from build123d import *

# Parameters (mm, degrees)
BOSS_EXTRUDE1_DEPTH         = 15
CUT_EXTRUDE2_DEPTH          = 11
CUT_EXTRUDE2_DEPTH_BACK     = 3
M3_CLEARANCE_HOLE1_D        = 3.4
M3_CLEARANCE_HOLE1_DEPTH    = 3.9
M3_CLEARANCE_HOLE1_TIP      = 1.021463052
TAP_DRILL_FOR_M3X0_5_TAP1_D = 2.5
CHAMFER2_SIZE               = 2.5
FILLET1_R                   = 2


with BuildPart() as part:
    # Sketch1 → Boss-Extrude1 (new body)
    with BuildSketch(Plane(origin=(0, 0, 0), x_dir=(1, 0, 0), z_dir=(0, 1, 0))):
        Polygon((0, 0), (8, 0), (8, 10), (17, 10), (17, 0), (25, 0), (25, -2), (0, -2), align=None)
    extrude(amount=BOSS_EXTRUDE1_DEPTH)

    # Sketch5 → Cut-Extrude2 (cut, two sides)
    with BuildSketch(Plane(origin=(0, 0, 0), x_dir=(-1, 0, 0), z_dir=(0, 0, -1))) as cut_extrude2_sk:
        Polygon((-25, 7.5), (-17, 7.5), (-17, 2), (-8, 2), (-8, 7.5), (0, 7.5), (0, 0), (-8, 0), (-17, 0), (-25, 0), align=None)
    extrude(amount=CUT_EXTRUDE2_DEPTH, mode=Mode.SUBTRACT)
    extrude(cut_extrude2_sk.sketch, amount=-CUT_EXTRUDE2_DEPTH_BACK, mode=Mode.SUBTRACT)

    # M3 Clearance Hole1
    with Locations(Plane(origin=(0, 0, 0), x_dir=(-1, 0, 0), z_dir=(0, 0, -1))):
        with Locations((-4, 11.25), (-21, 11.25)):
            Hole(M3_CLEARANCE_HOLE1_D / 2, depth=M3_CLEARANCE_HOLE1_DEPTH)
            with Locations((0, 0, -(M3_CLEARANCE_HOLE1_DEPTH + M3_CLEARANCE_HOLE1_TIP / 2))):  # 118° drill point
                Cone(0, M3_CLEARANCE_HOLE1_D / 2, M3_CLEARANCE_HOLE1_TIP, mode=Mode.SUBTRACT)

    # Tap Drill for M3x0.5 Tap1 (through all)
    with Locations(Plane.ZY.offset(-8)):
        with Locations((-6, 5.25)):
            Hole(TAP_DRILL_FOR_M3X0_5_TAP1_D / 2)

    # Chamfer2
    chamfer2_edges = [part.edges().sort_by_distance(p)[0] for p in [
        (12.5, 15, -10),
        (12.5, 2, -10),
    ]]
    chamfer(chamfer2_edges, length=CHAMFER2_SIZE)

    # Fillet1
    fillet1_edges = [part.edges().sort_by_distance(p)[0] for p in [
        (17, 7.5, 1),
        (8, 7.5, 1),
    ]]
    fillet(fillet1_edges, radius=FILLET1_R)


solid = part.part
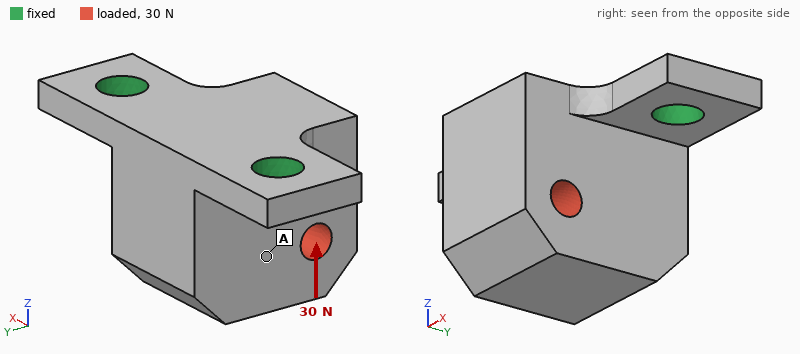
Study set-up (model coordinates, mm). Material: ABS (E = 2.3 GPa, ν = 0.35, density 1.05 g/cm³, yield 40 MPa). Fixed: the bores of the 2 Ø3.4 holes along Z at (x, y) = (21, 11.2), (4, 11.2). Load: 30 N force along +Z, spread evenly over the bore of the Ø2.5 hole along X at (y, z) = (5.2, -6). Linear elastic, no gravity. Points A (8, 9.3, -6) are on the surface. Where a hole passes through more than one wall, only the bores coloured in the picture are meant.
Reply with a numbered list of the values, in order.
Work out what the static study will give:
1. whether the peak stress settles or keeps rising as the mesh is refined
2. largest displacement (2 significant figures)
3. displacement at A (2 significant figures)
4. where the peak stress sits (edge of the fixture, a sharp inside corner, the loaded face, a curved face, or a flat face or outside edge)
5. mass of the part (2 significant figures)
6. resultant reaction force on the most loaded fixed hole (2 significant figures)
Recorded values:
1. keeps rising
2. 0.17 mm
3. 0.098 mm
4. edge of the fixture
5. 1.6 g
6. 16 N
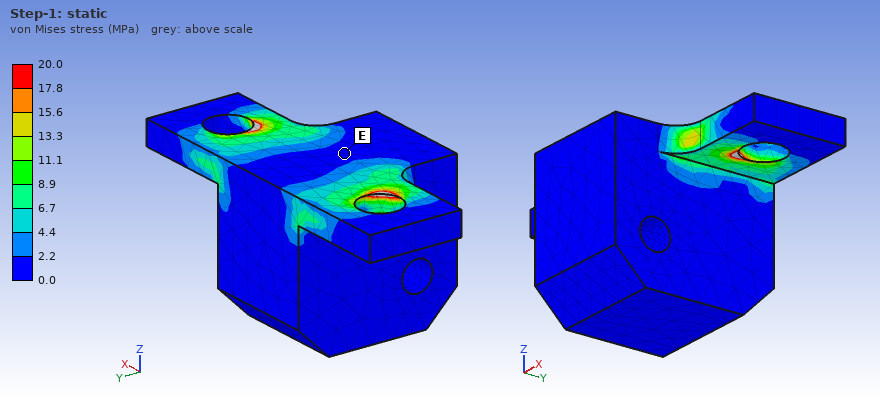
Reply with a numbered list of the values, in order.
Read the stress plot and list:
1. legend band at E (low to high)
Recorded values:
1. 0.0 to 2.2 MPa
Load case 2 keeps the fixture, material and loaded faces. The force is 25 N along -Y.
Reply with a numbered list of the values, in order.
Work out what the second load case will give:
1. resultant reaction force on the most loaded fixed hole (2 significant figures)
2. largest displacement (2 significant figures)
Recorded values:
1. 13 N
2. 0.17 mm
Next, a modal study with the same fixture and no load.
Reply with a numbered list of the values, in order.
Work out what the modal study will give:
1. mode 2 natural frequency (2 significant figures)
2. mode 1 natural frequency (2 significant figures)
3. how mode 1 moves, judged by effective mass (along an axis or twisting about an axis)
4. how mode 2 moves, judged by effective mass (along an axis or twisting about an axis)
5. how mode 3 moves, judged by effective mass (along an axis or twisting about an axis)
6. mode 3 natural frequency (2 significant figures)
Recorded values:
1. 5900 Hz
2. 2100 Hz
3. along Y
4. along X
5. along Z
6. 7100 Hz
